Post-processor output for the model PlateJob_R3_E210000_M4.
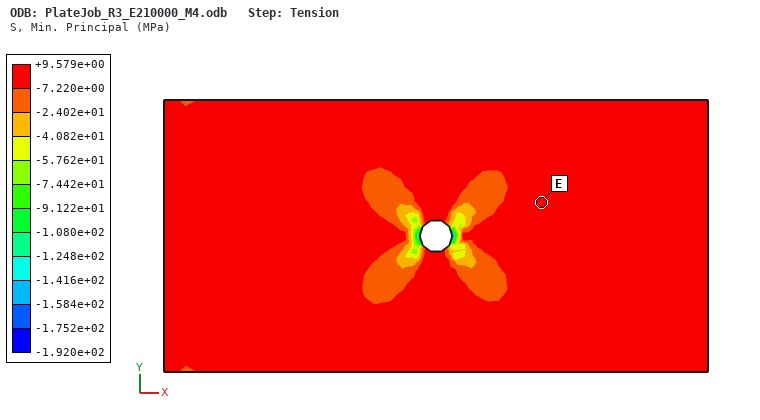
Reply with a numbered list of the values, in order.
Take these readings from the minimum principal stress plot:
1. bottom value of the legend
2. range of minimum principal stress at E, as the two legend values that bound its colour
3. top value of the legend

1. -1.920e+02 MPa
2. -7.220e+00 to +9.579e+00 MPa
3. +9.579e+00 MPa
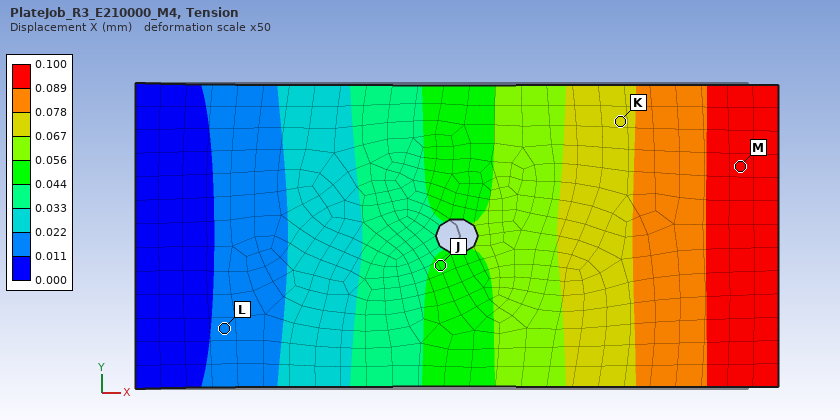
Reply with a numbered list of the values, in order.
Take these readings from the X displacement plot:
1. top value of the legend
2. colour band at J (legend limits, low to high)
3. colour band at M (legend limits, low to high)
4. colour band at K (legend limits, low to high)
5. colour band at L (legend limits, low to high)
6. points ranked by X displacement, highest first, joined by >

1. 0.100 mm
2. 0.044 to 0.056 mm
3. 0.089 to 0.100 mm
4. 0.067 to 0.078 mm
5. 0.011 to 0.022 mm
6. M > K > J > L
